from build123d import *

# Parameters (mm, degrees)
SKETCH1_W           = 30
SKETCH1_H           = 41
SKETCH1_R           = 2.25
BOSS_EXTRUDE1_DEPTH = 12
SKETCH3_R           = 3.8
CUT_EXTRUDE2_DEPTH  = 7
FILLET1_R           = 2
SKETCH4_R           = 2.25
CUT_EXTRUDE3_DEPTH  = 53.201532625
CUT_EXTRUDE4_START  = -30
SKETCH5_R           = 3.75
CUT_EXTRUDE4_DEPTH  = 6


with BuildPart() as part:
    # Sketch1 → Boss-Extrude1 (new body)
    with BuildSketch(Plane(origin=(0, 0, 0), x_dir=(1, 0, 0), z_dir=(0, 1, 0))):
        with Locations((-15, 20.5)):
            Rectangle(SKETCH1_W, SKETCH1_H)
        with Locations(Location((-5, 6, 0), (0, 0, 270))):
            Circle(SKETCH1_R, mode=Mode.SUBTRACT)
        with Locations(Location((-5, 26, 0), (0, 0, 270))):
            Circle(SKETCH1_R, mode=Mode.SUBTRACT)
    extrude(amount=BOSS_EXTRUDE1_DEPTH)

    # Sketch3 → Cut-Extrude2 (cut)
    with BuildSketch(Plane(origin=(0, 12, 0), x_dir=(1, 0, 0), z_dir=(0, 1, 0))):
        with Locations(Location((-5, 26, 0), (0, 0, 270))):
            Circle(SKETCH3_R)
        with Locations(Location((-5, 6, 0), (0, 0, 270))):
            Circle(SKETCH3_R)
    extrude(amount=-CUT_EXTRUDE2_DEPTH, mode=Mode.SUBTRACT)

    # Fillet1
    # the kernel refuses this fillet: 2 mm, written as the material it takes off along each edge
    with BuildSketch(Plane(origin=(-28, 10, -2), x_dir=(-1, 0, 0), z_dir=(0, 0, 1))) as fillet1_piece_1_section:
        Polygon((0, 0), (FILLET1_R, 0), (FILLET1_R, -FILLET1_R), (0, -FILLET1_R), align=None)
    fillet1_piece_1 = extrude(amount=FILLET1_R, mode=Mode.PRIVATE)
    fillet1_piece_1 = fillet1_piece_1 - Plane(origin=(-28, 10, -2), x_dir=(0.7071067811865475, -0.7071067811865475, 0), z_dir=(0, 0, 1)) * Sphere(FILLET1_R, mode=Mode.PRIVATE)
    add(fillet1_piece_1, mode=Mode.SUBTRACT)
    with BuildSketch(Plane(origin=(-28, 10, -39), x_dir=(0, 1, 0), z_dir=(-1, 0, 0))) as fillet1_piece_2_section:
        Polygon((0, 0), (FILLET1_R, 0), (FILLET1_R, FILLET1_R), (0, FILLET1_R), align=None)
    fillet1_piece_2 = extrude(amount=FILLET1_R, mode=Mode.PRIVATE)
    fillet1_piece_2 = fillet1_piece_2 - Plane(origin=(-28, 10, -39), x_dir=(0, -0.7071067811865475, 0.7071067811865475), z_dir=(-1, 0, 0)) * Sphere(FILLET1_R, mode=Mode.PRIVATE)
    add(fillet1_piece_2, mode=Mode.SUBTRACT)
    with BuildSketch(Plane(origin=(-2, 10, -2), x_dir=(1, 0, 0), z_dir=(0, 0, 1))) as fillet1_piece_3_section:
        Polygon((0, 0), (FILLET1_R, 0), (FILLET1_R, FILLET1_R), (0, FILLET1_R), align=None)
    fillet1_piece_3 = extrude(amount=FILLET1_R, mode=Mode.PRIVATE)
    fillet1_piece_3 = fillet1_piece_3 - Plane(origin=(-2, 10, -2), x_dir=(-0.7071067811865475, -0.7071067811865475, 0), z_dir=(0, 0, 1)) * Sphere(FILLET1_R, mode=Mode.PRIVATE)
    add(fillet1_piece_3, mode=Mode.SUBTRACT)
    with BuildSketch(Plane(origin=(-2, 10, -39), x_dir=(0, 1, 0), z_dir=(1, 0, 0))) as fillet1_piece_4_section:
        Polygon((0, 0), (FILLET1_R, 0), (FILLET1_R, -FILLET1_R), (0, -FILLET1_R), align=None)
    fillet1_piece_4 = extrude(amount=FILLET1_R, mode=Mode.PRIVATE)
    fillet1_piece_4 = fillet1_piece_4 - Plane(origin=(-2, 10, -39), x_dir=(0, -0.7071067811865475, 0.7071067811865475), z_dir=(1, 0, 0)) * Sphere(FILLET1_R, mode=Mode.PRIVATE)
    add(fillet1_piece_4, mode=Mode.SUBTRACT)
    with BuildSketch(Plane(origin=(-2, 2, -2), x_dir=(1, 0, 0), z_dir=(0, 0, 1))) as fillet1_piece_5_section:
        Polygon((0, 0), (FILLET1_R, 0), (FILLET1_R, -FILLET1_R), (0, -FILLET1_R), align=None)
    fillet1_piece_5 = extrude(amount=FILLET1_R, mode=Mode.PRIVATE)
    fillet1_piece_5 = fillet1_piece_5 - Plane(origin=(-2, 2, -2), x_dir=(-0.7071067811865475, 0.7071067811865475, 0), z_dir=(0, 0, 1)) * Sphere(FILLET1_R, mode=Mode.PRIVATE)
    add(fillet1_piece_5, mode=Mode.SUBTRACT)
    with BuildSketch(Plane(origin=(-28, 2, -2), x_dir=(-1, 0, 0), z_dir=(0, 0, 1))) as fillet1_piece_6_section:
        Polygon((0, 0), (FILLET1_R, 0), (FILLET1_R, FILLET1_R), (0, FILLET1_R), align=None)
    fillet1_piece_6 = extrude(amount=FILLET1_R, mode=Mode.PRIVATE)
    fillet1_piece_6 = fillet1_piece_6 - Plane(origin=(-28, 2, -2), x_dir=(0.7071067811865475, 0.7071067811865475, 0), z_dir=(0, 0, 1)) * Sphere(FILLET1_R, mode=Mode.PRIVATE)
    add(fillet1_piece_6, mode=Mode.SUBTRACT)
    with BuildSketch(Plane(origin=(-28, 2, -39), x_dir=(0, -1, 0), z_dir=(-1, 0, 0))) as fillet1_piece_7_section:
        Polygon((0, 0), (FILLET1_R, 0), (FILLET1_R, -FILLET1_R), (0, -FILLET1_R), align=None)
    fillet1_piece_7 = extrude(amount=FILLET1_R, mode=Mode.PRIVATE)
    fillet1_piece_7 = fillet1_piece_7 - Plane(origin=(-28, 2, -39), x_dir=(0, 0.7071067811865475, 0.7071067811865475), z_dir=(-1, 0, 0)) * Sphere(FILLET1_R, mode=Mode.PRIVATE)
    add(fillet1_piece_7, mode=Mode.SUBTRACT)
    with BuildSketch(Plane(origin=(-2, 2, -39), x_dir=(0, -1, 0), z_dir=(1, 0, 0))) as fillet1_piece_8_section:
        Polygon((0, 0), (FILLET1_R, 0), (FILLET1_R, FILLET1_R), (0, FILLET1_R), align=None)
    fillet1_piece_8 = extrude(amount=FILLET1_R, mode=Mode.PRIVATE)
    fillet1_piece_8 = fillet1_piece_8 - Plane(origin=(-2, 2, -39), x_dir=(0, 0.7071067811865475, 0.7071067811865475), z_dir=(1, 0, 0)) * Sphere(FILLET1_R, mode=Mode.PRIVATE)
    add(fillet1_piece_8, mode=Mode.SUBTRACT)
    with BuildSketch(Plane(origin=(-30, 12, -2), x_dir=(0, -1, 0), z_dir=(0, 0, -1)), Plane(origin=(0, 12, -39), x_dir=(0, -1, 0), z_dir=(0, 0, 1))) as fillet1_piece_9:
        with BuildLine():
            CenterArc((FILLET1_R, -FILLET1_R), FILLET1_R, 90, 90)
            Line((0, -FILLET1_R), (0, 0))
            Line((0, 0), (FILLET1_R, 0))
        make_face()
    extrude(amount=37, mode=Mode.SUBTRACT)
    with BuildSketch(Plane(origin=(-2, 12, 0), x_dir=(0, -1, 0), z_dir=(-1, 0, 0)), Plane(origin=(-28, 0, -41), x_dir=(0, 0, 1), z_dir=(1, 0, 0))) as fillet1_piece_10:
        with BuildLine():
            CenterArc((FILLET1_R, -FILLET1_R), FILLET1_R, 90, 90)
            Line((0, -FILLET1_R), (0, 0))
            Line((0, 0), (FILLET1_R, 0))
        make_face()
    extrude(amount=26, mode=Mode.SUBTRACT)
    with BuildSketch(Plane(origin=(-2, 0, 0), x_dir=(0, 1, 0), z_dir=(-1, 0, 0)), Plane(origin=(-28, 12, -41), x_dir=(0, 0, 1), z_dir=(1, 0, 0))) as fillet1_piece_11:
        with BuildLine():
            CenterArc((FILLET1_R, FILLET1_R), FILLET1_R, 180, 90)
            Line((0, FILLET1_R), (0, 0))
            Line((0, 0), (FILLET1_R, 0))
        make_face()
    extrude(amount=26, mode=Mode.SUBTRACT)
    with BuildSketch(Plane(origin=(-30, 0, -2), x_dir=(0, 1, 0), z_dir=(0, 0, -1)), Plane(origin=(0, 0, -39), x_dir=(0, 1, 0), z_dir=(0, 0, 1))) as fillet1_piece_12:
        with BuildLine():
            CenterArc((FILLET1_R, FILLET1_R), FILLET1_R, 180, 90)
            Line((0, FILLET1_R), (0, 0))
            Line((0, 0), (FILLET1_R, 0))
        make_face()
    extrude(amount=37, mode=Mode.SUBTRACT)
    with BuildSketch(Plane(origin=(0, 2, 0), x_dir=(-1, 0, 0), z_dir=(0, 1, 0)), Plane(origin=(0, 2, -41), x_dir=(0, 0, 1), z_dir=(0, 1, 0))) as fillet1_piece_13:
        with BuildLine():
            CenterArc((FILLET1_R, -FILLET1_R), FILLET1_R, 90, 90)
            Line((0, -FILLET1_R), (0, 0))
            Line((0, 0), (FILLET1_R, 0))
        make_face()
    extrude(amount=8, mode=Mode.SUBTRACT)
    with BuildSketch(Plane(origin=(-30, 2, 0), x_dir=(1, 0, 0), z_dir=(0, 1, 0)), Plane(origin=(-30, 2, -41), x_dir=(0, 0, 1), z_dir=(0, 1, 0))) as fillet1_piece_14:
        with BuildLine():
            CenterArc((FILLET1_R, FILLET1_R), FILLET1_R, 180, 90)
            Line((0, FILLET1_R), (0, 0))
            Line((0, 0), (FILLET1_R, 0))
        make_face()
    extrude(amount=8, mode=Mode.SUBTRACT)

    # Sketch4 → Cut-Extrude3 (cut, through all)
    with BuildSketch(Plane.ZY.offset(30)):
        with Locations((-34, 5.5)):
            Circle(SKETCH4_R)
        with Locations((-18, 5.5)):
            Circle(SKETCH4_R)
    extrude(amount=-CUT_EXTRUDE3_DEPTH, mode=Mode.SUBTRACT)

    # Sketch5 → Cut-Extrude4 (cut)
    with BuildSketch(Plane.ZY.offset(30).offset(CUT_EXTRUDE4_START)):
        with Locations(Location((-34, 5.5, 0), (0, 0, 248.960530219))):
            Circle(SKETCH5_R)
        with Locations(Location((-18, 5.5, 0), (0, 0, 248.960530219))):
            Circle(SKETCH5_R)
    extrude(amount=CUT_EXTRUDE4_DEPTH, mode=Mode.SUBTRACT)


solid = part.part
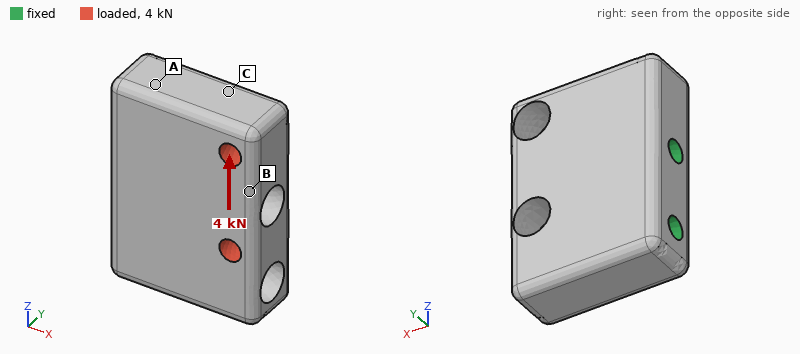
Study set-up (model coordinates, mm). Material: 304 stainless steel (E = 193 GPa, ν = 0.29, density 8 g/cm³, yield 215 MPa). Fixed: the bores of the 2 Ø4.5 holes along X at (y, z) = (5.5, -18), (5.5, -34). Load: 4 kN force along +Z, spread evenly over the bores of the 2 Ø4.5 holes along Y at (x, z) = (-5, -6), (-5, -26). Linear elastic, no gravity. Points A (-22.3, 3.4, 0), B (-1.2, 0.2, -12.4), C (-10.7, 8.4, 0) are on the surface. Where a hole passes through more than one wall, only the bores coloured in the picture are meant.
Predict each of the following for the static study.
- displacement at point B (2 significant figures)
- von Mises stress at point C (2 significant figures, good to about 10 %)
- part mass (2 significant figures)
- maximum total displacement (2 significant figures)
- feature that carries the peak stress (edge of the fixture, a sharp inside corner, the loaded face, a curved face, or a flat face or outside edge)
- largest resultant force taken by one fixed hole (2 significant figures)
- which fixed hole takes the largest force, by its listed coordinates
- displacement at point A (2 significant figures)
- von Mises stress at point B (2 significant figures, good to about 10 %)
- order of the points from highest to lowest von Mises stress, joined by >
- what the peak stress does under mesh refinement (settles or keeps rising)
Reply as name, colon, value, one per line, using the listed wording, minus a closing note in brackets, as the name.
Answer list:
displacement at point B: 3.3 µm
von Mises stress at point C: 17 MPa
part mass: 99 g
maximum total displacement: 5.3 µm
feature that carries the peak stress: edge of the fixture
largest resultant force taken by one fixed hole: 2.9 kN
which fixed hole takes the largest force, by its listed coordinates: (5.5, -18)
displacement at point A: 1.6 µm
von Mises stress at point B: 31 MPa
order of the points from highest to lowest von Mises stress, joined by >: B > C > A
what the peak stress does under mesh refinement: keeps rising
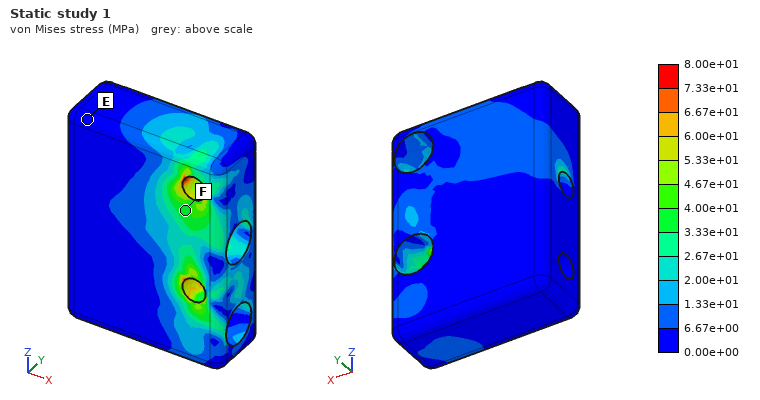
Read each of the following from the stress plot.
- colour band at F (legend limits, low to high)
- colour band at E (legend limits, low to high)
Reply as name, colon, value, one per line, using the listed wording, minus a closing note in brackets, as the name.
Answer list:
colour band at F: 3.33e+01 to 4.00e+01 MPa
colour band at E: 0.00e+00 to 6.67e+00 MPa
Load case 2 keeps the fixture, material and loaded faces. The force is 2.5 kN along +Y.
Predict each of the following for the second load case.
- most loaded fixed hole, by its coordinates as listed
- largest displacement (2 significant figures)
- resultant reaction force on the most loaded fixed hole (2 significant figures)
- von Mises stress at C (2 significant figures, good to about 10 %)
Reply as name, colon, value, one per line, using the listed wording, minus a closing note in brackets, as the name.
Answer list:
most loaded fixed hole, by its coordinates as listed: (5.5, -18)
largest displacement: 6.9 µm
resultant reaction force on the most loaded fixed hole: 2.2 kN
von Mises stress at C: 13 MPa
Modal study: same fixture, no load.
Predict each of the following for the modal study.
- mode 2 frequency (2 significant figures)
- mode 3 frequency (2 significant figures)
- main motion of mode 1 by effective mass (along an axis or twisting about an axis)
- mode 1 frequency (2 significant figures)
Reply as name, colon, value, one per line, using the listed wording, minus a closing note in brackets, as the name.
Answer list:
mode 2 frequency: 30 kHz
mode 3 frequency: 31 kHz
main motion of mode 1 by effective mass: along Y
mode 1 frequency: 20 kHz
